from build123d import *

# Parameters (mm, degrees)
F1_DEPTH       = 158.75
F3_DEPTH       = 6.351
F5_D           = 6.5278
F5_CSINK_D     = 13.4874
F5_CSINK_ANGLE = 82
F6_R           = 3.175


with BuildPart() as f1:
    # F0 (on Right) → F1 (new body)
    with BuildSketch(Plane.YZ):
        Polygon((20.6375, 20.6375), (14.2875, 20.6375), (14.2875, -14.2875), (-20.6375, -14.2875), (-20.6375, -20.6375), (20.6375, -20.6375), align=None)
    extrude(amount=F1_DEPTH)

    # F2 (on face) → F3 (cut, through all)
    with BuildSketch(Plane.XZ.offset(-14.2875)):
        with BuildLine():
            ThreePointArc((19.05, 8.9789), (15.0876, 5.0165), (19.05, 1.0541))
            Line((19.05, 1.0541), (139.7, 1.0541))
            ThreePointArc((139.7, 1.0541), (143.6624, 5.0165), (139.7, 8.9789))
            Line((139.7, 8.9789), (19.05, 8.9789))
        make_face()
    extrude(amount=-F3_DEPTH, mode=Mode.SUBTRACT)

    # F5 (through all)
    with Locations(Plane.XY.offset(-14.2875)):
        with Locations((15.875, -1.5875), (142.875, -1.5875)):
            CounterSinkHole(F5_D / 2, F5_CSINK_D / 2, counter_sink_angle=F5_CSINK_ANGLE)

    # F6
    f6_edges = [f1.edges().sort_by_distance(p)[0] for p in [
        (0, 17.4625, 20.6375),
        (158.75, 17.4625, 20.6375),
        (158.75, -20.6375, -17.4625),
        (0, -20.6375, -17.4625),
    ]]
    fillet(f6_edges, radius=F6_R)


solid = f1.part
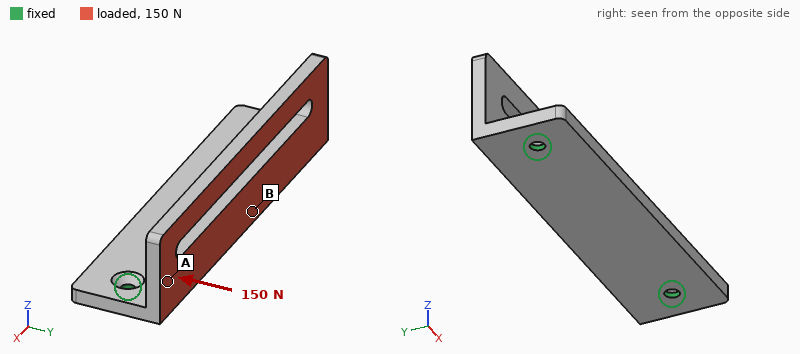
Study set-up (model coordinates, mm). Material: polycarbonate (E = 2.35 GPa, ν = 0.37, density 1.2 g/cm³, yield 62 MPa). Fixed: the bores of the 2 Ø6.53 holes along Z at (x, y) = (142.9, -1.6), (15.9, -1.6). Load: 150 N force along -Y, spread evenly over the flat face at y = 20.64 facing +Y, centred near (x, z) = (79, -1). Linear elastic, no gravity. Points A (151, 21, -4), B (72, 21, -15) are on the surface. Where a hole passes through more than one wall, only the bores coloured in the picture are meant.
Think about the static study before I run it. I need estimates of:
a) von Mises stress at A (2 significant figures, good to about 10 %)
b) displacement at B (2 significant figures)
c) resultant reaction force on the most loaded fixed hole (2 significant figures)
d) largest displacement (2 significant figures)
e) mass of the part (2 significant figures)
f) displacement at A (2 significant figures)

3.9 MPa
0.38 mm
77 N
1.9 mm
83 g
0.49 mm
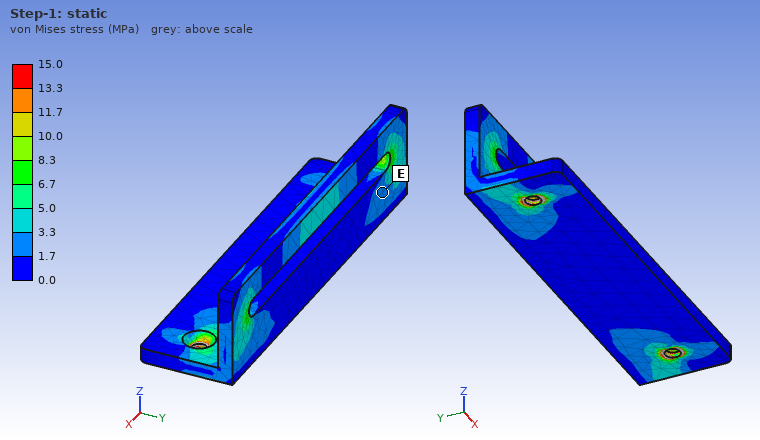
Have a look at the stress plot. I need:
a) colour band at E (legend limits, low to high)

1.7 to 3.3 MPa
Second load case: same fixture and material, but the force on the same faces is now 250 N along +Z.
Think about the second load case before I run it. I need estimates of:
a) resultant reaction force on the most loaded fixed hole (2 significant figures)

130 N
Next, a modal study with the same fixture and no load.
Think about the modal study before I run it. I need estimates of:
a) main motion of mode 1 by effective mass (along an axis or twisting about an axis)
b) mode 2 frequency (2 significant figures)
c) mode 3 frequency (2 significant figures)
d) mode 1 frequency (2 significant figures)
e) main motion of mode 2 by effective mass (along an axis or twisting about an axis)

along Y
500 Hz
530 Hz
260 Hz
along Z
